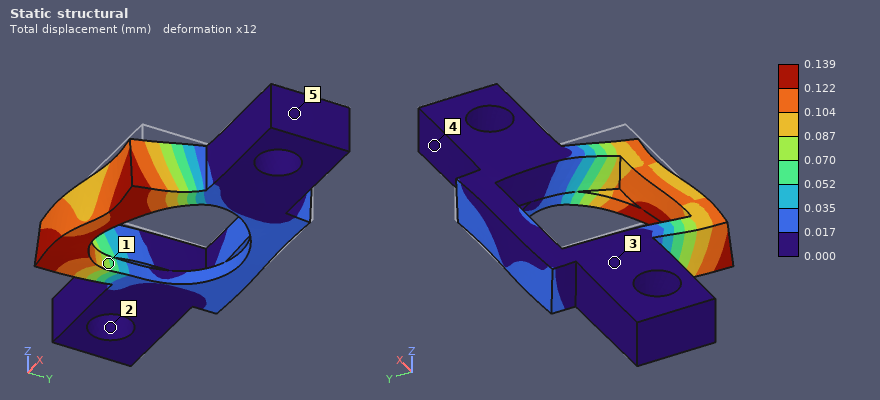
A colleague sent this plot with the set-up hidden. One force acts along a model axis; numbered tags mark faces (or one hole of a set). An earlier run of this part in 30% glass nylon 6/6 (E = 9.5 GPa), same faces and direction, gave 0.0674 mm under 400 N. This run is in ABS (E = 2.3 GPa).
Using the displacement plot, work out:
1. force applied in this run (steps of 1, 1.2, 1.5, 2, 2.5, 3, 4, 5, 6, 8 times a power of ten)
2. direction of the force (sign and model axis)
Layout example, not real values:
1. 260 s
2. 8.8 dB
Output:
1. 200 N
2. -X
